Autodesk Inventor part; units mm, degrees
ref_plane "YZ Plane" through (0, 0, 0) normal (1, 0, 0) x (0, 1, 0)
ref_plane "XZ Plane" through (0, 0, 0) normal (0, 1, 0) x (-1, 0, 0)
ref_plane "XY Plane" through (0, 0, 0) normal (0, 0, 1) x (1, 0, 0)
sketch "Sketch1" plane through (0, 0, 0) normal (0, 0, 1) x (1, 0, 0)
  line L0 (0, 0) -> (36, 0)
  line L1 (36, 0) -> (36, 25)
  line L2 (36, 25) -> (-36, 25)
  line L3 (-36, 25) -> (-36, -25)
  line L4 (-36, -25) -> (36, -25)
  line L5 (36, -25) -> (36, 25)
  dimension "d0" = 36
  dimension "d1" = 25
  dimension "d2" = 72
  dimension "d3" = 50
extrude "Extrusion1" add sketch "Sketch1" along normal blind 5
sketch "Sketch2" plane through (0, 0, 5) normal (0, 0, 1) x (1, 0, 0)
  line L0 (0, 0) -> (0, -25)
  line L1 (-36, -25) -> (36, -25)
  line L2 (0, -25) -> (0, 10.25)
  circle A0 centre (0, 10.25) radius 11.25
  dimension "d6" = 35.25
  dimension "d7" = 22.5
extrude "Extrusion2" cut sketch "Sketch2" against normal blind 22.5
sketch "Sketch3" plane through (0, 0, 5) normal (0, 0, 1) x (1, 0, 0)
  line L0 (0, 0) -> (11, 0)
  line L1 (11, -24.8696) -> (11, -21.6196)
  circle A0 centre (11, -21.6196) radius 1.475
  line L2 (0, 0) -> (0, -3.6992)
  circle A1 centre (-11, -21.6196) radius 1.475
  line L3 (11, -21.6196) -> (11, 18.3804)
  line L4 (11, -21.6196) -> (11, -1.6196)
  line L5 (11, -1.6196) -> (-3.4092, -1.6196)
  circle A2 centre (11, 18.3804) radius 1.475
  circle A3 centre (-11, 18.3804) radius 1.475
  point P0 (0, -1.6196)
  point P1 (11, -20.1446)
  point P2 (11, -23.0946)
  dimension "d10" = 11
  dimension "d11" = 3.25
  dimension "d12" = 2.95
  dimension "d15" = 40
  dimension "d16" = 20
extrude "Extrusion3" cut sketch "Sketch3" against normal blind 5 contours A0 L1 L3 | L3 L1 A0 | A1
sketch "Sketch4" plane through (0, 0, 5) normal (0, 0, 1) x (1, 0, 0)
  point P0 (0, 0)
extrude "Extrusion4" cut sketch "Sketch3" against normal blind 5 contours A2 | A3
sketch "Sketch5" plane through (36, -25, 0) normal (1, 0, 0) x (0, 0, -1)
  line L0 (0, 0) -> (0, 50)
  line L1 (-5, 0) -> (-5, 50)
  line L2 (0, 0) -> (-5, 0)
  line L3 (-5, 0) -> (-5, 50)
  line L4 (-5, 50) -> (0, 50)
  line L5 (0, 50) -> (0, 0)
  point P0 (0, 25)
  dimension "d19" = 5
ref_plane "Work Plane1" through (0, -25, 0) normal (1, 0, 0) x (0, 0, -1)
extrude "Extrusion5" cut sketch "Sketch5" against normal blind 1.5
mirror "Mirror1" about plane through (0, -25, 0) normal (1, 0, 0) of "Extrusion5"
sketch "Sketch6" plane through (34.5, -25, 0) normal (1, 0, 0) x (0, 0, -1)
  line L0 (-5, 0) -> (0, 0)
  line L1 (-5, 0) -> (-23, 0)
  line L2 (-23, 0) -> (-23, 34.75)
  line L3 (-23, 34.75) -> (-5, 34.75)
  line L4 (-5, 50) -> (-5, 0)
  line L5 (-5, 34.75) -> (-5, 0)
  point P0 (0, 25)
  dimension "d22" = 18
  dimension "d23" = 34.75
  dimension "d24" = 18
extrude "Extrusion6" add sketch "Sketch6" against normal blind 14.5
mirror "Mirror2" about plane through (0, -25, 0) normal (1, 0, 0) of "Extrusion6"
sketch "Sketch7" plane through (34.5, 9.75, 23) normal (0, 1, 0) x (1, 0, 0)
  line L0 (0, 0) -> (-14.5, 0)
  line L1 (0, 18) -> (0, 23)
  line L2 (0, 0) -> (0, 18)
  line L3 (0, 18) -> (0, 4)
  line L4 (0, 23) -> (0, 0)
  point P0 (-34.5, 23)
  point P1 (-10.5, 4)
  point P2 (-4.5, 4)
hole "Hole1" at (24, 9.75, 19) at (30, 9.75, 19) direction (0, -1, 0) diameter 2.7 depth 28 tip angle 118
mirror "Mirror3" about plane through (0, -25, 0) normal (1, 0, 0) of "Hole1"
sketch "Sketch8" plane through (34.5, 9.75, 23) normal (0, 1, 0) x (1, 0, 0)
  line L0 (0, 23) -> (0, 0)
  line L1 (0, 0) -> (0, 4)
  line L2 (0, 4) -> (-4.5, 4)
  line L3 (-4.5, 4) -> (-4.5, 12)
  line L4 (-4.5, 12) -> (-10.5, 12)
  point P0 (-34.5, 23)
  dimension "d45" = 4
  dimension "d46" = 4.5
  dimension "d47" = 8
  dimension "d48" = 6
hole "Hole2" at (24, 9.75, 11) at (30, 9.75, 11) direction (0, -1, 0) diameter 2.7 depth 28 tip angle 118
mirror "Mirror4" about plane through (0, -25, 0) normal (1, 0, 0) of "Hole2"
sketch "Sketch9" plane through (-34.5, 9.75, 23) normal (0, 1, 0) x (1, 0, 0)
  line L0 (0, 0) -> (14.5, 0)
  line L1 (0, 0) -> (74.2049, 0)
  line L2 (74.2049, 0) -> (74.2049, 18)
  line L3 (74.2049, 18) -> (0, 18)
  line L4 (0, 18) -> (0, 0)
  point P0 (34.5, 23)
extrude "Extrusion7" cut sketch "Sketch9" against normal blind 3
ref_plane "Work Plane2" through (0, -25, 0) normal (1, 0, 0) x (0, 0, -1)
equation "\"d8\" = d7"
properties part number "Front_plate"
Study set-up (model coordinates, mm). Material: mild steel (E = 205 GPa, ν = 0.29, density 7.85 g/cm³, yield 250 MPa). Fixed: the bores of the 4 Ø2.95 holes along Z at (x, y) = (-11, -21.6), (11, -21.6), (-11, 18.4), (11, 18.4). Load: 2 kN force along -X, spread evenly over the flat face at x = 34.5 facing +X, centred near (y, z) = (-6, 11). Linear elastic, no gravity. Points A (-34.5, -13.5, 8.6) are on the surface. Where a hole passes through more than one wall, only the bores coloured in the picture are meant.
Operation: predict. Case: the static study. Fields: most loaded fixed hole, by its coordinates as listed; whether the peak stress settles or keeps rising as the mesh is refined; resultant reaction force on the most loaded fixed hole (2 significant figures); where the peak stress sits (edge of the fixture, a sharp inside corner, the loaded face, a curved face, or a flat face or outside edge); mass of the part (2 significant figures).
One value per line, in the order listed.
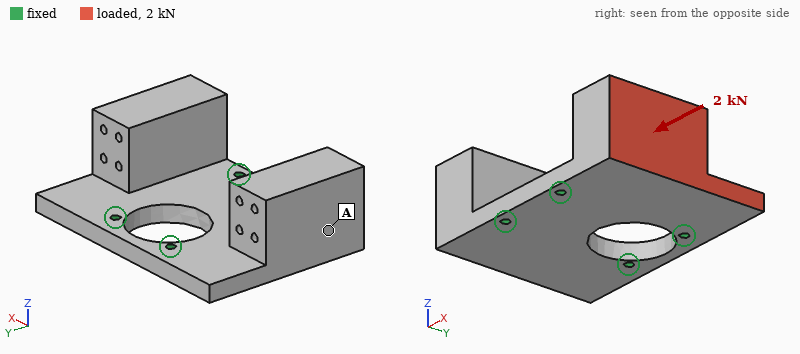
(11, -21.6)
keeps rising
1000 N
edge of the fixture
240 g
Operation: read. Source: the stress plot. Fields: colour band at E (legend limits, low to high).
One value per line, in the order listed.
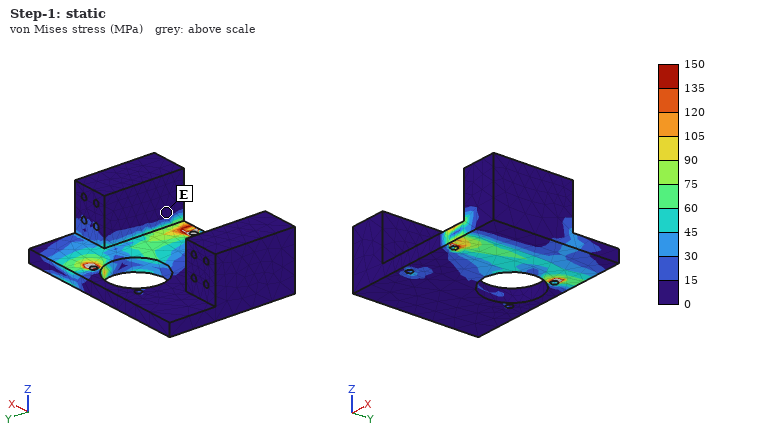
0 to 15 MPa
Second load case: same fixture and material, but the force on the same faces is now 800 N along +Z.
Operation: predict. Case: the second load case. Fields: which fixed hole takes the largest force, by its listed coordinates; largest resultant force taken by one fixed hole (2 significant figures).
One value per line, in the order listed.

(11, -21.6)
680 N
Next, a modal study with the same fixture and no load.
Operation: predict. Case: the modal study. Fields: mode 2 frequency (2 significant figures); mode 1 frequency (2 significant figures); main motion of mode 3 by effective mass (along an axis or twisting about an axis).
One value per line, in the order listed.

2700 Hz
2600 Hz
along Y
